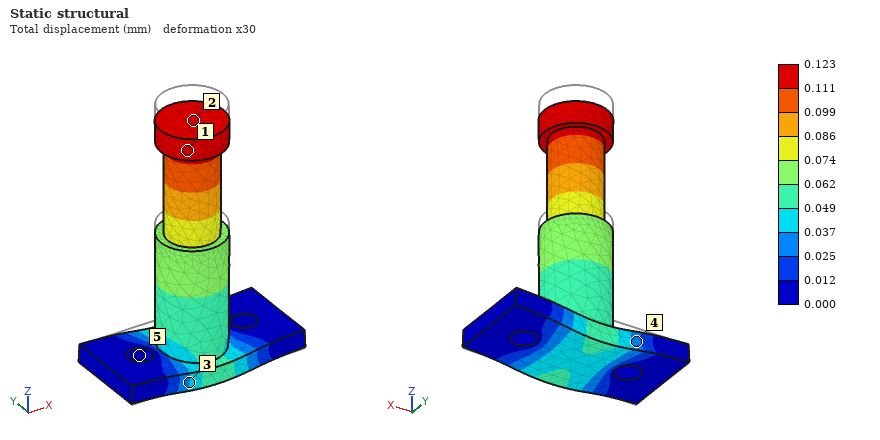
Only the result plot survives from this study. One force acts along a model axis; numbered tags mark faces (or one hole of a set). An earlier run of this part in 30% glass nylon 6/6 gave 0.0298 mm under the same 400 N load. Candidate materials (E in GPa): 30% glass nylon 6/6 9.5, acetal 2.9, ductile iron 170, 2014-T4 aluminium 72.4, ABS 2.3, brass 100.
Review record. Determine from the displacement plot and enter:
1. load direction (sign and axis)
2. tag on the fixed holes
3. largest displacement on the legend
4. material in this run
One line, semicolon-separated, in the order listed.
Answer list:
-Z; 5; 0.123 mm; ABS
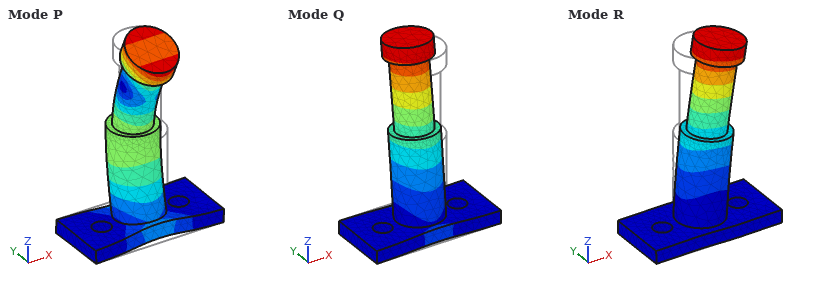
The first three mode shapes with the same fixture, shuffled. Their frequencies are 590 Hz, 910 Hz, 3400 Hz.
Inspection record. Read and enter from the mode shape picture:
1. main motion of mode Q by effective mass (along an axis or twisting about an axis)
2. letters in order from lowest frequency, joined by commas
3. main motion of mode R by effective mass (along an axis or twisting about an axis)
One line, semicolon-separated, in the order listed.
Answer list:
along Y; Q, R, P; along X
